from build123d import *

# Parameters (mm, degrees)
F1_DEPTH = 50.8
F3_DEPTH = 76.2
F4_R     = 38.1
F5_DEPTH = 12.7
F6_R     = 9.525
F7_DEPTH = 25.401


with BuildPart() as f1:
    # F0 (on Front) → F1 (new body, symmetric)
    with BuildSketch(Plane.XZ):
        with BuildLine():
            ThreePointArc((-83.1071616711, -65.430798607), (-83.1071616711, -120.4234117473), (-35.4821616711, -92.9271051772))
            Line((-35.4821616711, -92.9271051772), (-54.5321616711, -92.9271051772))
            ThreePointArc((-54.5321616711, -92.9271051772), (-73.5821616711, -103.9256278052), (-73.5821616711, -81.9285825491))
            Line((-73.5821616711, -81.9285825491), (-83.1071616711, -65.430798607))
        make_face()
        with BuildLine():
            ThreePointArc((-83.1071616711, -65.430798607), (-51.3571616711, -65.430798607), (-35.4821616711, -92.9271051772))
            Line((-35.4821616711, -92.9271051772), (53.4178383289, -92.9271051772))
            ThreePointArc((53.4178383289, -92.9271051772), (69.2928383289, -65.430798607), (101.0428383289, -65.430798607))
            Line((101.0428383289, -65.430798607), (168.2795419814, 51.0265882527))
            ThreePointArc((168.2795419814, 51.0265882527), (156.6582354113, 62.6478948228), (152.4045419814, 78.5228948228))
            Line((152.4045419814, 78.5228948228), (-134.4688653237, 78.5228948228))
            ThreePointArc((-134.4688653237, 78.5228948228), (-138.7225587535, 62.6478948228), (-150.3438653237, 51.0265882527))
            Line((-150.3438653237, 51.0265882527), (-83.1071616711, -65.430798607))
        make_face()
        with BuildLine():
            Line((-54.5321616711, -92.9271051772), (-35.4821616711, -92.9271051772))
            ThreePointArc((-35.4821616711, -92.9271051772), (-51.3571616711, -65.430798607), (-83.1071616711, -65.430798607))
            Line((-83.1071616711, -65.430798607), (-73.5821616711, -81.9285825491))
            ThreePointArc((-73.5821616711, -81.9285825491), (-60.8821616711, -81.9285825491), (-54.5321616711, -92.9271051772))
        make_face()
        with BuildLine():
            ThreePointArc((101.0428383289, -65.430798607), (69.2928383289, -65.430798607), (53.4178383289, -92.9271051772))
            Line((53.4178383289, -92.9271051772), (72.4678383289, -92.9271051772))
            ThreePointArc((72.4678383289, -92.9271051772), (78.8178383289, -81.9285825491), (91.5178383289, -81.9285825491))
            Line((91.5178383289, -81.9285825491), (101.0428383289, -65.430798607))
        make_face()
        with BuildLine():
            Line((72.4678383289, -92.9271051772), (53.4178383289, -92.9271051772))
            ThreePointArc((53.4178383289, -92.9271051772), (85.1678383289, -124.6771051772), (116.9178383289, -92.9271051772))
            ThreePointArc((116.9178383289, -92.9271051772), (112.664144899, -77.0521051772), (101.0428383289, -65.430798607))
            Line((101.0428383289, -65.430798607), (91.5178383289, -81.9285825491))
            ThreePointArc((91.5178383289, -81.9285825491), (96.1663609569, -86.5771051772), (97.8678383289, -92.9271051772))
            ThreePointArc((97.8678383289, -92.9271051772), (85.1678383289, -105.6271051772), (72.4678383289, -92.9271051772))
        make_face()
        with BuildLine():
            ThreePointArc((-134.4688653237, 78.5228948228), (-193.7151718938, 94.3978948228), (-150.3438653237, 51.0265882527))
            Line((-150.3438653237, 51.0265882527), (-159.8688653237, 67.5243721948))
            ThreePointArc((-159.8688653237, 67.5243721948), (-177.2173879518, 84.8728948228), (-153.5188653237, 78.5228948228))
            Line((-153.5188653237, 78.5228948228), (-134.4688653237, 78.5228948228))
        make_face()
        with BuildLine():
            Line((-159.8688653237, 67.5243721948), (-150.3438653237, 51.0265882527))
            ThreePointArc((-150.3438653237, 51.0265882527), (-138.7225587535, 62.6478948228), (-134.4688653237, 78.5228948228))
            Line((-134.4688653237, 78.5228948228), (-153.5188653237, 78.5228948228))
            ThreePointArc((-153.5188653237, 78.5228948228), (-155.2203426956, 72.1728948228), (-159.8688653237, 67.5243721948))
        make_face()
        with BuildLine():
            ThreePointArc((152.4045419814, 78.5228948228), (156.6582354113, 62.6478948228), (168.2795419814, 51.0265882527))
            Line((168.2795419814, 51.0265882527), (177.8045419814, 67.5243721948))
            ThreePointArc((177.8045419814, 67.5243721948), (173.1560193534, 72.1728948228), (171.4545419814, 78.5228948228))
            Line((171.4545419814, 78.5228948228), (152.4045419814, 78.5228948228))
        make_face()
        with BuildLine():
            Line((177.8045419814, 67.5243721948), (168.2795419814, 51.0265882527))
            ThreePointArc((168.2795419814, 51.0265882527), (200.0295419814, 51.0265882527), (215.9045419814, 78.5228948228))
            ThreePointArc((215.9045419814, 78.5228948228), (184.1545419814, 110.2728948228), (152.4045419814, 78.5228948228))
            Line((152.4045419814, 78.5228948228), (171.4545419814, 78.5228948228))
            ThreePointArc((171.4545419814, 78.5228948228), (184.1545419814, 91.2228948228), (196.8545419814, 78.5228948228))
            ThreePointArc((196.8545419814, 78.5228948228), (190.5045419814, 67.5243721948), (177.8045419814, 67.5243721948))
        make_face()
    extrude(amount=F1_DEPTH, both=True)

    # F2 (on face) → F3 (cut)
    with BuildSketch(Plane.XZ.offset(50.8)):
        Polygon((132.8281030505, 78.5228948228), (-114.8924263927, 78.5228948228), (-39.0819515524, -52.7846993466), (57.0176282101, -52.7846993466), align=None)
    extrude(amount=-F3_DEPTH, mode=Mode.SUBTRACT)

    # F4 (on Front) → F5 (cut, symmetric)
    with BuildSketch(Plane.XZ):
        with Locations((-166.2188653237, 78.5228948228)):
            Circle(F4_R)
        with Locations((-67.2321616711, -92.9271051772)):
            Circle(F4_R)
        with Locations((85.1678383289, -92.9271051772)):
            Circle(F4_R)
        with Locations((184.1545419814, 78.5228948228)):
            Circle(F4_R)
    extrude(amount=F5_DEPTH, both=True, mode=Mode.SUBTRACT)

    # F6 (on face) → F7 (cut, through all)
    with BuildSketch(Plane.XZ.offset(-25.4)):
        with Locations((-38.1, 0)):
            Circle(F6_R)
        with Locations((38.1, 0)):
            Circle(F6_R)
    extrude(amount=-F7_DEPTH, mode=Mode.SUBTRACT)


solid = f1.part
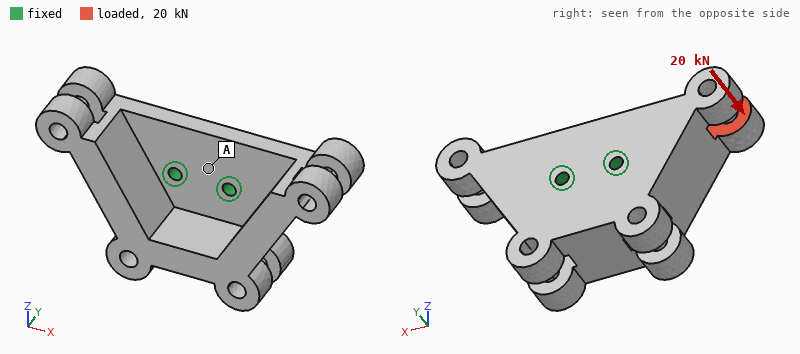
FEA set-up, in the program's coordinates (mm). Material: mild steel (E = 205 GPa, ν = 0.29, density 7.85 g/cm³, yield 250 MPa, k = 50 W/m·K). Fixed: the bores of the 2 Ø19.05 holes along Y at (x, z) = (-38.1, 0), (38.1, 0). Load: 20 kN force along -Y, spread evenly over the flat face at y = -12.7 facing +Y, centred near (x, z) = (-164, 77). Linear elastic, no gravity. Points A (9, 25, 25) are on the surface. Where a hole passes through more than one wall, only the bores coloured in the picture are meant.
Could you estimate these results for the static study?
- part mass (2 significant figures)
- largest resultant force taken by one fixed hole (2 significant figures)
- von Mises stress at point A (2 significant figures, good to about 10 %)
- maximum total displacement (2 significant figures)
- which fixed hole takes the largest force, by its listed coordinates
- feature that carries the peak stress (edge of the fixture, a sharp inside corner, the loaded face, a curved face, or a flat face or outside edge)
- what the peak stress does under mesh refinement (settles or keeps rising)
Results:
24 kg
39 kN
13 MPa
0.30 mm
(-38.1, 0)
edge of the fixture
keeps rising
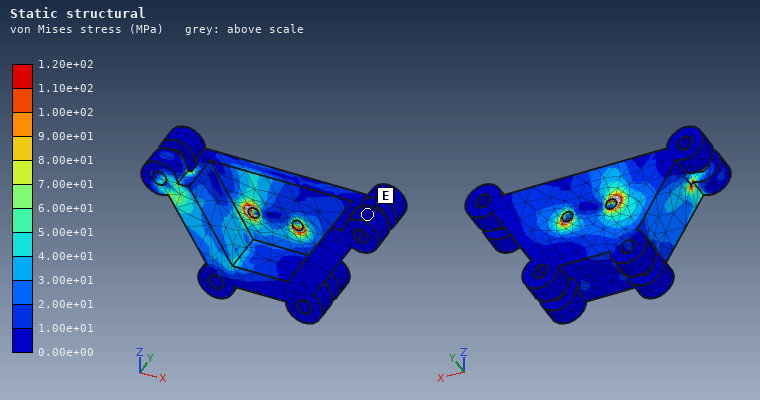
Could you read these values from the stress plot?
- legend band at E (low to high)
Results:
0.00e+00 to 1.00e+01 MPa
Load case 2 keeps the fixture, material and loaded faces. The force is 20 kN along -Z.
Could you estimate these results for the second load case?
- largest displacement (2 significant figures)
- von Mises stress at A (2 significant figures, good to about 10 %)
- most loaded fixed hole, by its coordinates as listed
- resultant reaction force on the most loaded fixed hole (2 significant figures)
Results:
0.19 mm
12 MPa
(-38.1, 0)
46 kN
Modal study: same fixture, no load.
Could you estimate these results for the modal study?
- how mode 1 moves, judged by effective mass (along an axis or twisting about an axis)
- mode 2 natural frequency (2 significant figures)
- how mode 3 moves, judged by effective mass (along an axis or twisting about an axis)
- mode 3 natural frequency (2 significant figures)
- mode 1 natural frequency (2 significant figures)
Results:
along Z
760 Hz
twisting about Y
1200 Hz
670 Hz
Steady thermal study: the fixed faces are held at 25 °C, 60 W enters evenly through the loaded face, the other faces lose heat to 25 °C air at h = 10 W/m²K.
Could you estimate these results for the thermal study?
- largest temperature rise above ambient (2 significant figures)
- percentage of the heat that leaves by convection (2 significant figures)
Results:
69 K
38 %
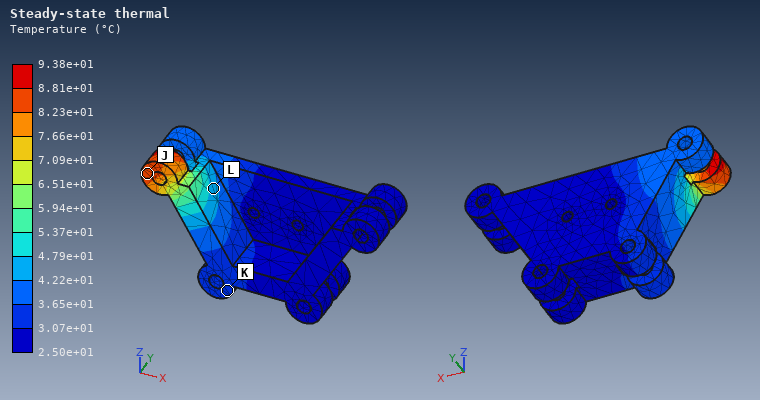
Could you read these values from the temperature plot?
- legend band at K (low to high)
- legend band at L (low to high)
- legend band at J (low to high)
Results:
3.07e+01 to 3.65e+01 °C
4.22e+01 to 4.79e+01 °C
8.23e+01 to 8.81e+01 °C
